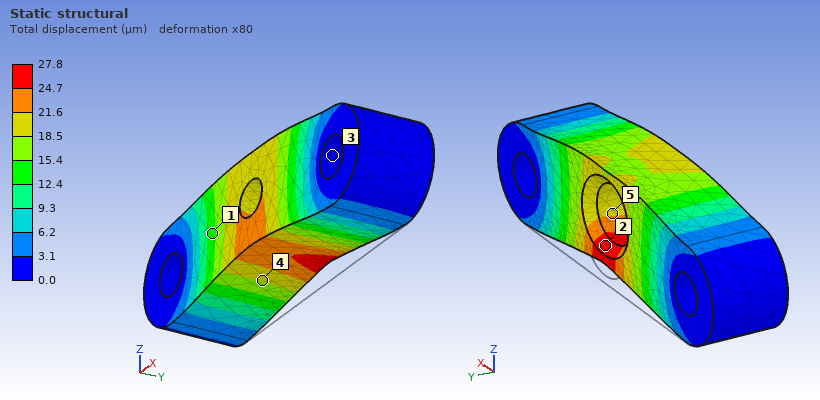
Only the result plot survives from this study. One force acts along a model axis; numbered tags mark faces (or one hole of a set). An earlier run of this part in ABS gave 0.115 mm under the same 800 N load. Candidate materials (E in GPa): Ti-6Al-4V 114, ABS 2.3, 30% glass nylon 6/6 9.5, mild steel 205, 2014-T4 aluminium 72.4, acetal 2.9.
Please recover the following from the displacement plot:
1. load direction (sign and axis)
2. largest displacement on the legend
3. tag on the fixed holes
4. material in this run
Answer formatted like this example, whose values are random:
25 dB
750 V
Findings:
+Z
27.8 µm
3
30% glass nylon 6/6
